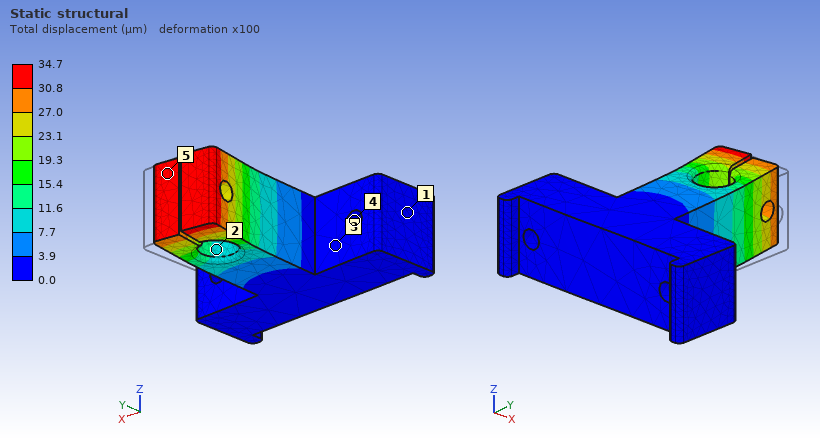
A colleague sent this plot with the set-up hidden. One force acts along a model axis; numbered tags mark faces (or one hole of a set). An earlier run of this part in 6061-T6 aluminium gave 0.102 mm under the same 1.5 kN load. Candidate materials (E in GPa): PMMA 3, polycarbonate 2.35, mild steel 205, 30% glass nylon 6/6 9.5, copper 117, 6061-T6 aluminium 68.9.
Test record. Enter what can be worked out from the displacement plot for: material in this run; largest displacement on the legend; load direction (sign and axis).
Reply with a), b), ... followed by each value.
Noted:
a) mild steel
b) 34.7 µm
c) -X
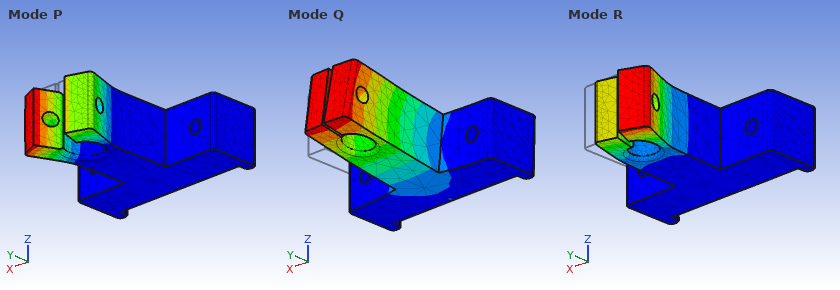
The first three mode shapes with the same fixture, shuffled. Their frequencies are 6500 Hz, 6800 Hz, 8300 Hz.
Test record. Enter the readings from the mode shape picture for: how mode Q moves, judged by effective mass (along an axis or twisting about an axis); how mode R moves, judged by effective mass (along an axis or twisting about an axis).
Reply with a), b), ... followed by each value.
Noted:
a) along Z
b) along X
